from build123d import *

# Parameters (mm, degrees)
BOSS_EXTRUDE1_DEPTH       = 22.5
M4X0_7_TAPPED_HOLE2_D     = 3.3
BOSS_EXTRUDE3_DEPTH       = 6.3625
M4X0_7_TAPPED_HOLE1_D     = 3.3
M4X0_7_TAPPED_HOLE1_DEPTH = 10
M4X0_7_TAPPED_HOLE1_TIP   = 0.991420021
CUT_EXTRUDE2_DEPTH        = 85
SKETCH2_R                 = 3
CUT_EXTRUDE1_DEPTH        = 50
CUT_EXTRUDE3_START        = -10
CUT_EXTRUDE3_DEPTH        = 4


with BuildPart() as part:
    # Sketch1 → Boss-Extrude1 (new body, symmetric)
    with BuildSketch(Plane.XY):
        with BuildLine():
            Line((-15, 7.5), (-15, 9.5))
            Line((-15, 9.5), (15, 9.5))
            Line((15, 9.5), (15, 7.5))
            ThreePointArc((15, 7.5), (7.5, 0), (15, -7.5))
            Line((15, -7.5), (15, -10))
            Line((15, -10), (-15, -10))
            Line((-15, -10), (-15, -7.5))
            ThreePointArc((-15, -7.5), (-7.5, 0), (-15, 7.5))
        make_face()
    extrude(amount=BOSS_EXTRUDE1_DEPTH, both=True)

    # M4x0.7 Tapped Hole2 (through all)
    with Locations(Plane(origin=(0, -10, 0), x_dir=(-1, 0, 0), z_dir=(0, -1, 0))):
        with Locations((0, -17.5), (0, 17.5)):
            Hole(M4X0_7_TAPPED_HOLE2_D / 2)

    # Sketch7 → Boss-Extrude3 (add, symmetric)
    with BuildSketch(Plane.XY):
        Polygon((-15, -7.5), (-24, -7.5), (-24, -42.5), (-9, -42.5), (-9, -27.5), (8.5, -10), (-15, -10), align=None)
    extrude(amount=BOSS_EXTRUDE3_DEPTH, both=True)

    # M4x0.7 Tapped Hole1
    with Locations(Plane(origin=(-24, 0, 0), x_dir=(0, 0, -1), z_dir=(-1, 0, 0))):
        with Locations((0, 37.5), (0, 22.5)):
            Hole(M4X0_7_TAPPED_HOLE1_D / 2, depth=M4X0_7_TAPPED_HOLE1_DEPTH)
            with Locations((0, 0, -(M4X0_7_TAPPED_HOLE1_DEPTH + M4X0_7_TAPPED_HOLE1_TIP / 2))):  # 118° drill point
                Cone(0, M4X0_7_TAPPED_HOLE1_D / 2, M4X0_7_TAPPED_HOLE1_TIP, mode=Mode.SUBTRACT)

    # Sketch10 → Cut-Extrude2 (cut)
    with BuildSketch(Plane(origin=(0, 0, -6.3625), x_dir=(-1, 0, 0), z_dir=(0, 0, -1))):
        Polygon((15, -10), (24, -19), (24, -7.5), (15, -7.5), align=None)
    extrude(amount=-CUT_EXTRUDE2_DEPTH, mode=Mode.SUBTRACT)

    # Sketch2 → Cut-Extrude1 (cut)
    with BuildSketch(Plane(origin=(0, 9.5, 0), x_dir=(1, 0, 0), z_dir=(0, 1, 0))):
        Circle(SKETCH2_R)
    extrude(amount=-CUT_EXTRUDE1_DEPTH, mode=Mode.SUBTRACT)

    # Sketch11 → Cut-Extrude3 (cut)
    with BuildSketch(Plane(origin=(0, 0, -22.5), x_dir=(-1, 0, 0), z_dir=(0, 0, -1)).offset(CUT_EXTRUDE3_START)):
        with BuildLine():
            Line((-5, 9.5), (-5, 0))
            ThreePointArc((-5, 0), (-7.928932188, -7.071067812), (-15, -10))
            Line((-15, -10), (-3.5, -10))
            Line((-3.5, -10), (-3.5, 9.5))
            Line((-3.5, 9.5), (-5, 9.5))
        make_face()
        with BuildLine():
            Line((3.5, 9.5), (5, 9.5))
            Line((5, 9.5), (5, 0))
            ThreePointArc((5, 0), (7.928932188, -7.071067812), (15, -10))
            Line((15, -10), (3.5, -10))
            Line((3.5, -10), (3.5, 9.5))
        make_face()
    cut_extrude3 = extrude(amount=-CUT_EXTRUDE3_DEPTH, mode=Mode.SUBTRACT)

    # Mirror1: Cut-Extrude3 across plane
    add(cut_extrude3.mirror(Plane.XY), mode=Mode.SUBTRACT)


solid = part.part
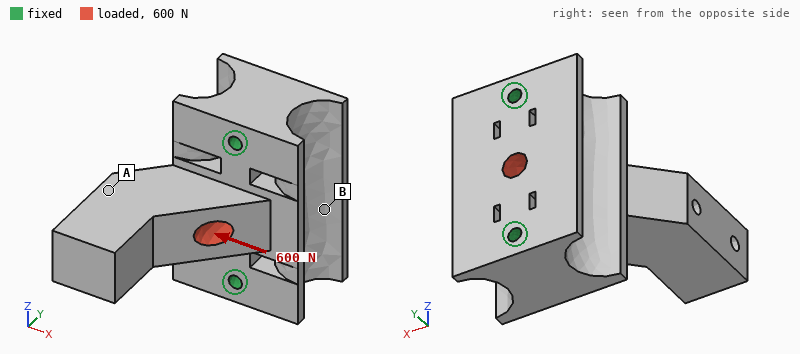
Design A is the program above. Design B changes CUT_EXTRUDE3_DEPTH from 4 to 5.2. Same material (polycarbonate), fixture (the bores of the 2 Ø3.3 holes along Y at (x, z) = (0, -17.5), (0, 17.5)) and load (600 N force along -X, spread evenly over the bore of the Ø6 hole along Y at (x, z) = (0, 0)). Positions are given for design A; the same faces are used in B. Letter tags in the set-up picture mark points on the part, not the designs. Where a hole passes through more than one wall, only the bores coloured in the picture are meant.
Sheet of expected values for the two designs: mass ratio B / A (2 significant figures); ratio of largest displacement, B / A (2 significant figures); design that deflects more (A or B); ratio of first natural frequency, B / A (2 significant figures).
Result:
0.99
1.1
B
0.97
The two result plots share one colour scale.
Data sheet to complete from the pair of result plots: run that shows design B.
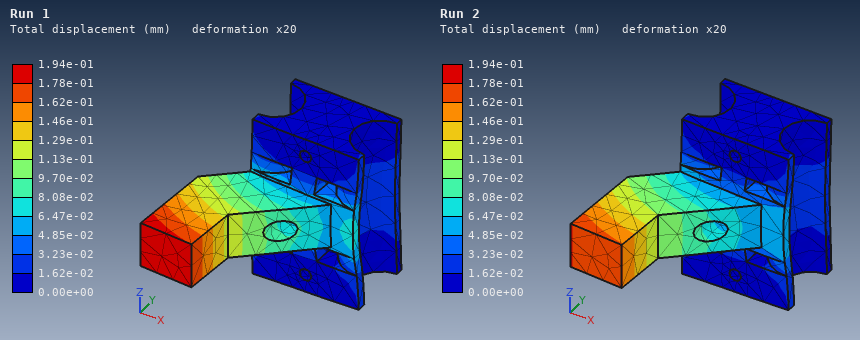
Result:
Run 1
